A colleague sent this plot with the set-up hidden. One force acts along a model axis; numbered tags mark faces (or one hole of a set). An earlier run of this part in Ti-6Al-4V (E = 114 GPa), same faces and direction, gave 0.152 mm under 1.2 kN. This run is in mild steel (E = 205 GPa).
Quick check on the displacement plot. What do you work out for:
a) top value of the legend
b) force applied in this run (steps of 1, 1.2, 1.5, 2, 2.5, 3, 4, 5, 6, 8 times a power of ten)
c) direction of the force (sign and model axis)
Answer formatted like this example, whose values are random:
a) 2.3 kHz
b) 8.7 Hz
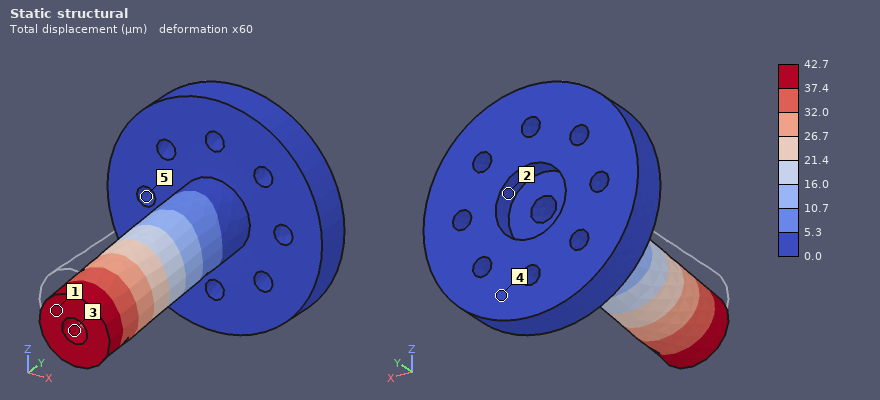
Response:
a) 42.7 µm
b) 600 N
c) -Z
